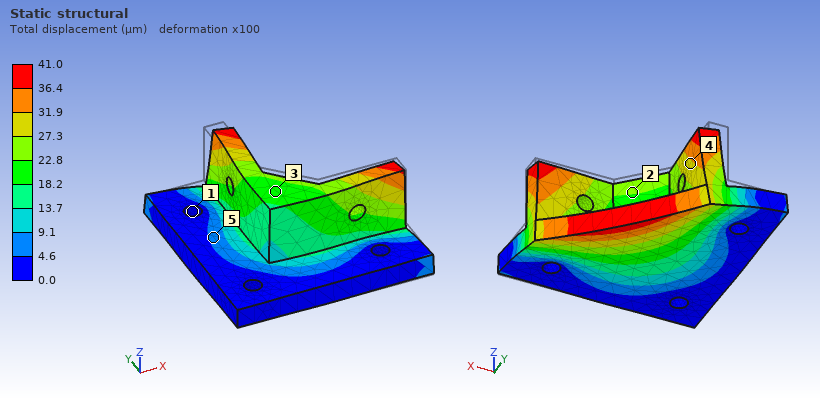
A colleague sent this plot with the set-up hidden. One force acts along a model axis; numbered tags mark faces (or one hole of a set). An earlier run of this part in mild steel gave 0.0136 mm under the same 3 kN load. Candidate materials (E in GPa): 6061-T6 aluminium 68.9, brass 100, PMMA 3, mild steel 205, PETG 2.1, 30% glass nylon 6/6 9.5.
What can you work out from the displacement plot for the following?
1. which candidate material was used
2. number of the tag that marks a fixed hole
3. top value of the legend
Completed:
6061-T6 aluminium
1
41.0 µm
